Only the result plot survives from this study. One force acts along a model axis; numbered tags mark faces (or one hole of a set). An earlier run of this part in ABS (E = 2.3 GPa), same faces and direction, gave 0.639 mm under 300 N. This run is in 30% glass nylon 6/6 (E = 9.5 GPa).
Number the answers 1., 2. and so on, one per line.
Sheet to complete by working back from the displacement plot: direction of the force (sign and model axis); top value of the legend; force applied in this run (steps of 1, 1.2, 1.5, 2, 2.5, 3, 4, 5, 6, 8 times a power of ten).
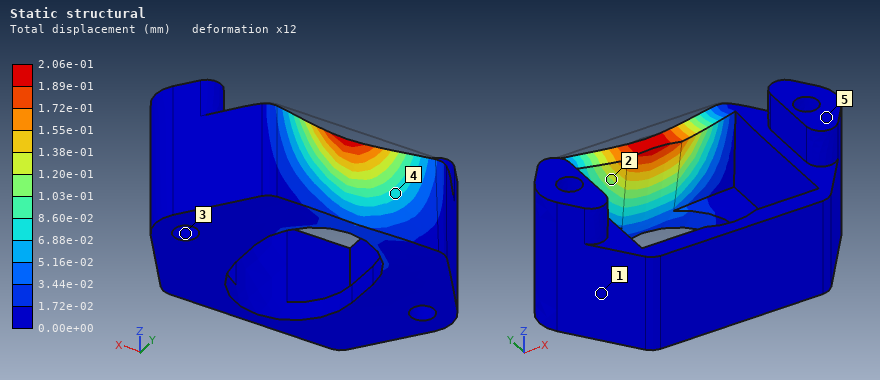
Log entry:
1. -Y
2. 2.06e-01 mm
3. 400 N
